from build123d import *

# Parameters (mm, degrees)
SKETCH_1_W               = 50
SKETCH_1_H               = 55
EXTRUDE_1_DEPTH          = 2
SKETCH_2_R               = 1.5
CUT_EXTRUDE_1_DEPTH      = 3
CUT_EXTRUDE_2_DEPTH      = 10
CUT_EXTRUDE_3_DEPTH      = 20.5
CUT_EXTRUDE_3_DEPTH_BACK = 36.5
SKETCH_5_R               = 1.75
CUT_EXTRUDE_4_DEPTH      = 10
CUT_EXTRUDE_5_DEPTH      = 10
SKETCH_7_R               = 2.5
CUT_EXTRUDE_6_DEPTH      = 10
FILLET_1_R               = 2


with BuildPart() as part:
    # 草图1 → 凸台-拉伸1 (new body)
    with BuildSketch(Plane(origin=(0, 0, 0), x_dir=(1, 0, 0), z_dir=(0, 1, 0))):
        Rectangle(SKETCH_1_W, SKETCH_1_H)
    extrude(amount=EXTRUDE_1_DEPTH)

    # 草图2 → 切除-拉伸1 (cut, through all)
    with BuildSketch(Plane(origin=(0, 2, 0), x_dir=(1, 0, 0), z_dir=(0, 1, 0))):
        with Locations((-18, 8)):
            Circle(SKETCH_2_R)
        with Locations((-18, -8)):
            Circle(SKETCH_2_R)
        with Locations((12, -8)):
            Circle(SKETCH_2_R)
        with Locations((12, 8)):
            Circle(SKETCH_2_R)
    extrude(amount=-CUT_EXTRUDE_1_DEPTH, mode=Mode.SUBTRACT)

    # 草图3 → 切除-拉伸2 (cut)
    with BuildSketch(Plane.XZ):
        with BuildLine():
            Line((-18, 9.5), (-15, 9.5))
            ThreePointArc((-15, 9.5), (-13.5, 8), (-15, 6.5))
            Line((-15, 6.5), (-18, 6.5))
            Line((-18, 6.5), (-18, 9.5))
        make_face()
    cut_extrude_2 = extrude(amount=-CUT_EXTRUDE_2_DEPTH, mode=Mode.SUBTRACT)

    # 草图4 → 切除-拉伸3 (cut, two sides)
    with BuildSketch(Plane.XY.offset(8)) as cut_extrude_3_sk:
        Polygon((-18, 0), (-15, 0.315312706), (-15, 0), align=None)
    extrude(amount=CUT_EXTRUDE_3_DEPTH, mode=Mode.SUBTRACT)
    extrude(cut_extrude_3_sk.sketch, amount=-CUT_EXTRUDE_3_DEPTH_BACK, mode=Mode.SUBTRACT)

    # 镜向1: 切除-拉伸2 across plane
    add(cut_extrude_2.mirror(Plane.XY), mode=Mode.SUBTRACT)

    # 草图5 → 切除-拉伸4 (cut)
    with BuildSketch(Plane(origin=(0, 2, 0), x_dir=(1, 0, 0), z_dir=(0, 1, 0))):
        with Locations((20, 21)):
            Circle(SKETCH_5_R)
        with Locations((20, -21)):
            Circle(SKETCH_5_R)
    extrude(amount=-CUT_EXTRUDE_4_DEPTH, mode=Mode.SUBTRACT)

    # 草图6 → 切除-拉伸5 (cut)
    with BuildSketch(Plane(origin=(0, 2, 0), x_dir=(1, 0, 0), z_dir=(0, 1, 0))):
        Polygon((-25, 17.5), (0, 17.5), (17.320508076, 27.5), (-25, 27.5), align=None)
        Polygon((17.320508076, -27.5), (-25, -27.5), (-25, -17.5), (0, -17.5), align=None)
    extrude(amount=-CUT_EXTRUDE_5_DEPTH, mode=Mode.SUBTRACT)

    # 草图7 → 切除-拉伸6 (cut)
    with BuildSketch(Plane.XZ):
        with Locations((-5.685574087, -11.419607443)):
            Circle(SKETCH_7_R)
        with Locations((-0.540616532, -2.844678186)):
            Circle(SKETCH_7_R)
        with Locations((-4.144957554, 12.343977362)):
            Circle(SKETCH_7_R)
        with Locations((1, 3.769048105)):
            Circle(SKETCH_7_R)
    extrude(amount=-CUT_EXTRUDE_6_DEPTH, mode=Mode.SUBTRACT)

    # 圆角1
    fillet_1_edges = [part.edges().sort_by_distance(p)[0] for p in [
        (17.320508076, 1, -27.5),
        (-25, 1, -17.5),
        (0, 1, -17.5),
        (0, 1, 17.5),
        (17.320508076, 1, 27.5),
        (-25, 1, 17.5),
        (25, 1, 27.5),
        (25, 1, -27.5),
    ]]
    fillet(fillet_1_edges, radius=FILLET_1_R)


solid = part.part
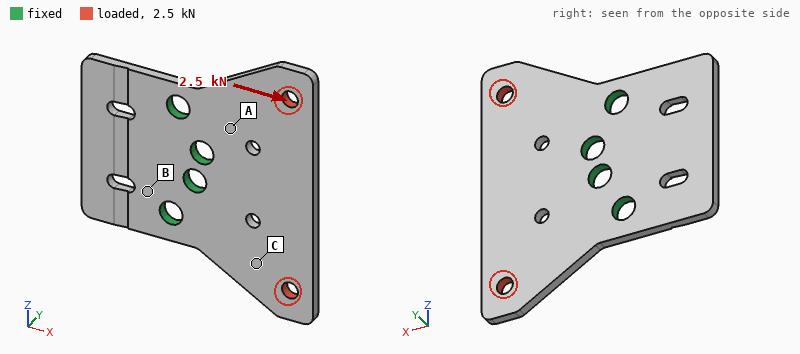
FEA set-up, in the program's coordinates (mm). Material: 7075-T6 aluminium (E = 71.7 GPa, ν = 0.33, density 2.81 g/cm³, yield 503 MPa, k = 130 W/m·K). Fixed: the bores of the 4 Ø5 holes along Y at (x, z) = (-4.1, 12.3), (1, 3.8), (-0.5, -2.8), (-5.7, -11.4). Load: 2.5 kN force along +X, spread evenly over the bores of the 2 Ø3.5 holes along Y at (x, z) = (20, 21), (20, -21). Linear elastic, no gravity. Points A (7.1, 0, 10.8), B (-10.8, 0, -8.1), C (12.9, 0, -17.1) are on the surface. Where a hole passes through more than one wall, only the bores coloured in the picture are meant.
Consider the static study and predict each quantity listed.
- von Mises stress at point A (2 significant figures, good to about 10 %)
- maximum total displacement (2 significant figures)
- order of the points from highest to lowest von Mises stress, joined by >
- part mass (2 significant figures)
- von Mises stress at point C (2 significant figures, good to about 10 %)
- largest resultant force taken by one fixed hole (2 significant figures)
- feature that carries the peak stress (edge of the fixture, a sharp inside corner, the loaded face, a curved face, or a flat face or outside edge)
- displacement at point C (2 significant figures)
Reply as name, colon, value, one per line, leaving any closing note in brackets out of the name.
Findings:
von Mises stress at point A: 34 MPa
maximum total displacement: 32 µm
order of the points from highest to lowest von Mises stress, joined by >: C > A > B
part mass: 11 g
von Mises stress at point C: 54 MPa
largest resultant force taken by one fixed hole: 900 N
feature that carries the peak stress: the loaded face
displacement at point C: 14 µm
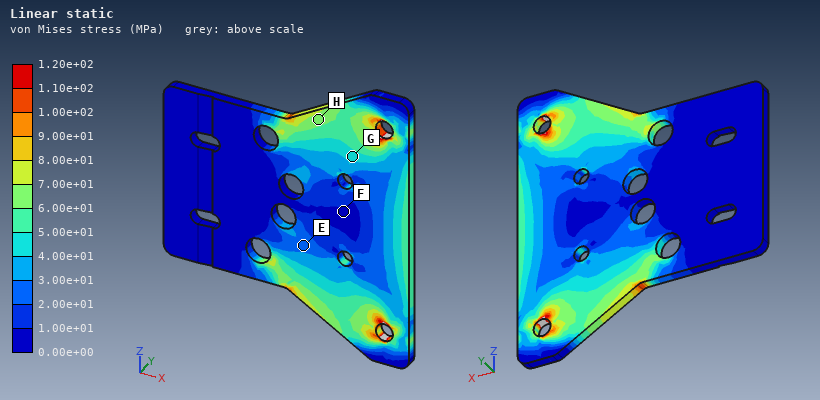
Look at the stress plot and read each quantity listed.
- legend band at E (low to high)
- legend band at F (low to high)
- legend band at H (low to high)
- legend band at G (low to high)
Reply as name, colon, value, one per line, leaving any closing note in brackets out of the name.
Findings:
legend band at E: 2.00e+01 to 3.00e+01 MPa
legend band at F: 0.00e+00 to 1.00e+01 MPa
legend band at H: 6.00e+01 to 7.00e+01 MPa
legend band at G: 4.00e+01 to 5.00e+01 MPa
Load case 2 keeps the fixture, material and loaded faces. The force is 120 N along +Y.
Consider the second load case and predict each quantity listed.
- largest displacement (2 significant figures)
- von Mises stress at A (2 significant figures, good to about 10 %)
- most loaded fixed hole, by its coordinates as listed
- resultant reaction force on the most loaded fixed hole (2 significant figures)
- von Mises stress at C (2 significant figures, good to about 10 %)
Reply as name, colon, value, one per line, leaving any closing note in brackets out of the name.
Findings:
largest displacement: 0.34 mm
von Mises stress at A: 56 MPa
most loaded fixed hole, by its coordinates as listed: (1, 3.8)
resultant reaction force on the most loaded fixed hole: 80 N
von Mises stress at C: 30 MPa
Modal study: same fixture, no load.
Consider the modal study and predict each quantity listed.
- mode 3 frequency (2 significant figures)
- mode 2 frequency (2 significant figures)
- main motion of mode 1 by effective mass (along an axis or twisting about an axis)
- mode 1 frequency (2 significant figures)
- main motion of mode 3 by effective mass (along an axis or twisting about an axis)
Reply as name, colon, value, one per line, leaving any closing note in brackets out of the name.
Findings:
mode 3 frequency: 4500 Hz
mode 2 frequency: 2700 Hz
main motion of mode 1 by effective mass: along Y
mode 1 frequency: 2300 Hz
main motion of mode 3 by effective mass: along Y
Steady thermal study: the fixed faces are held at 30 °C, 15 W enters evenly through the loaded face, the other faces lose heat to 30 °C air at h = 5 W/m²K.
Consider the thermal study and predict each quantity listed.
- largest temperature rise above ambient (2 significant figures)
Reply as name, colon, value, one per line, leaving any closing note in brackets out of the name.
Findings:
largest temperature rise above ambient: 44 K
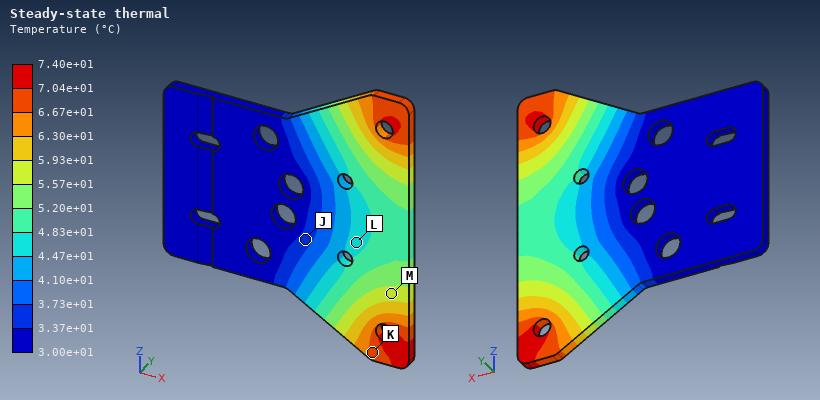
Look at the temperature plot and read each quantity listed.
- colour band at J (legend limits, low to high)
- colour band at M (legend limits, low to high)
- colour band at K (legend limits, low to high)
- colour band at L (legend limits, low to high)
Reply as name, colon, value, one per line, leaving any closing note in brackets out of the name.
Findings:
colour band at J: 3.37e+01 to 3.73e+01 °C
colour band at M: 5.57e+01 to 5.93e+01 °C
colour band at K: 6.67e+01 to 7.04e+01 °C
colour band at L: 4.47e+01 to 4.83e+01 °C
